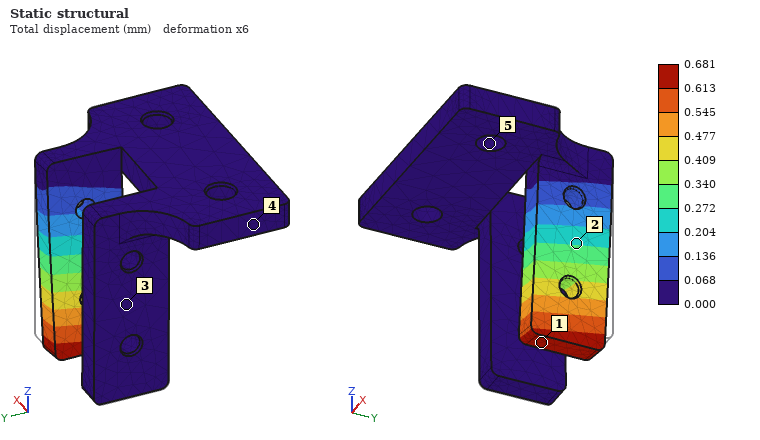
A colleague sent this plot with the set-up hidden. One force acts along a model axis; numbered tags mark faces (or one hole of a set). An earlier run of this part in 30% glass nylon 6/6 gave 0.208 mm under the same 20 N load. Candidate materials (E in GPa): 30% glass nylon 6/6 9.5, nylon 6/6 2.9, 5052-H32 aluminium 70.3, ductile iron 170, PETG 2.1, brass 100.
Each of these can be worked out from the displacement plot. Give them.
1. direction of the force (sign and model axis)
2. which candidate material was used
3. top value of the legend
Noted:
-X
nylon 6/6
0.681 mm
